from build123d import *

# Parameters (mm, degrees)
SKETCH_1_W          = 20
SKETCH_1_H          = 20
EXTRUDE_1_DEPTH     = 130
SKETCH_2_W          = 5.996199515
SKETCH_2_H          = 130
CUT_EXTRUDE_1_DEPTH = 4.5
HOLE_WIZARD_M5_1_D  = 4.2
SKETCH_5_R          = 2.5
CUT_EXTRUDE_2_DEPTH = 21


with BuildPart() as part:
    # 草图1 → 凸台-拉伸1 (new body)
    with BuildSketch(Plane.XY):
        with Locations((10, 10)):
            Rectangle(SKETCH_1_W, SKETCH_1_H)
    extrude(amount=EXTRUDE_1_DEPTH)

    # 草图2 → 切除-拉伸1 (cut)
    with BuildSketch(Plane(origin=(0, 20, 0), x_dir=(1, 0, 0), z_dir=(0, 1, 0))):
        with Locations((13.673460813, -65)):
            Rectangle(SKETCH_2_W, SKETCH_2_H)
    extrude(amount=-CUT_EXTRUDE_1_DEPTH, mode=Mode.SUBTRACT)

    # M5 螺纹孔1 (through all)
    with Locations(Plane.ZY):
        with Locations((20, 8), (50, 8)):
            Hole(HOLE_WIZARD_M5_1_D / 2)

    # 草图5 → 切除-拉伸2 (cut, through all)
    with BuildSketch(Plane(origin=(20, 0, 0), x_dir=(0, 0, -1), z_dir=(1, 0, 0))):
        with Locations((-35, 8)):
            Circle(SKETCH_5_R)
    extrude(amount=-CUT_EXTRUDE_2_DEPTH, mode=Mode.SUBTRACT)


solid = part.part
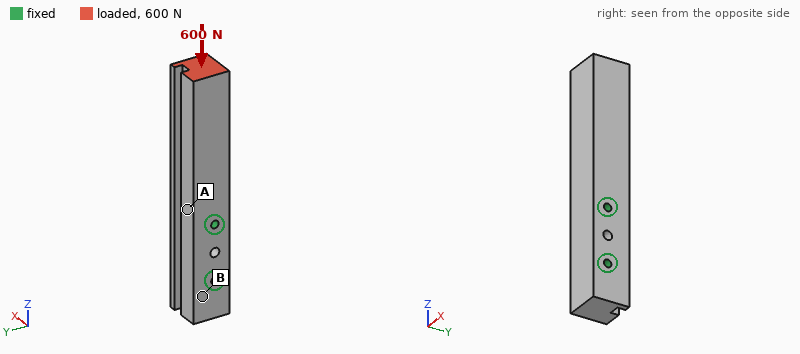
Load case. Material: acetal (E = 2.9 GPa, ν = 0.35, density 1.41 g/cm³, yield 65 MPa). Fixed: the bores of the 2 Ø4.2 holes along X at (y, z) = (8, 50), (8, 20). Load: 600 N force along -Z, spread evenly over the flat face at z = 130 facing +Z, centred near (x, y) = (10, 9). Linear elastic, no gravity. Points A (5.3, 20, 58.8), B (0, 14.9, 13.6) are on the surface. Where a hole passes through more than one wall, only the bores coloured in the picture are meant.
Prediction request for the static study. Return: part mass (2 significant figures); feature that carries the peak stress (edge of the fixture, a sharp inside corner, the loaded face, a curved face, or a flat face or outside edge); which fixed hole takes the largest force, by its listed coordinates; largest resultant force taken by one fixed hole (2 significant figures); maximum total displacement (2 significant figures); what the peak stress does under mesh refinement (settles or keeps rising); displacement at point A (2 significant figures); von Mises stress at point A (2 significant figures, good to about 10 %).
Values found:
67 g
edge of the fixture
(8, 50)
530 N
55 µm
keeps rising
11 µm
1.3 MPa
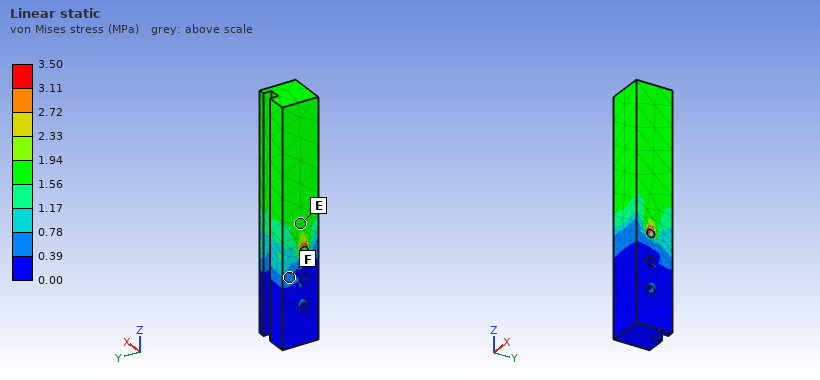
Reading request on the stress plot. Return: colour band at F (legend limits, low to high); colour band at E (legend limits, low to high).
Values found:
0.39 to 0.78 MPa
1.56 to 1.94 MPa
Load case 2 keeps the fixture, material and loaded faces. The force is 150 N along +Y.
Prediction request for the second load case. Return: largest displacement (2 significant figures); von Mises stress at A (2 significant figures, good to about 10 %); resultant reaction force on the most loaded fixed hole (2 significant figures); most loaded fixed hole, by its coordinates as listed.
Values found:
1.1 mm
9.6 MPa
450 N
(8, 50)
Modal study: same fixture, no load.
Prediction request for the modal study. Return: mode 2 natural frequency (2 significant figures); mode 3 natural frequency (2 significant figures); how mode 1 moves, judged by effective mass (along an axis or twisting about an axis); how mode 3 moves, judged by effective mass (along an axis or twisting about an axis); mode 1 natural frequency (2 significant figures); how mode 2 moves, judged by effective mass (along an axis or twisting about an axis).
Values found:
670 Hz
2200 Hz
along Y
twisting about Z
560 Hz
along X
